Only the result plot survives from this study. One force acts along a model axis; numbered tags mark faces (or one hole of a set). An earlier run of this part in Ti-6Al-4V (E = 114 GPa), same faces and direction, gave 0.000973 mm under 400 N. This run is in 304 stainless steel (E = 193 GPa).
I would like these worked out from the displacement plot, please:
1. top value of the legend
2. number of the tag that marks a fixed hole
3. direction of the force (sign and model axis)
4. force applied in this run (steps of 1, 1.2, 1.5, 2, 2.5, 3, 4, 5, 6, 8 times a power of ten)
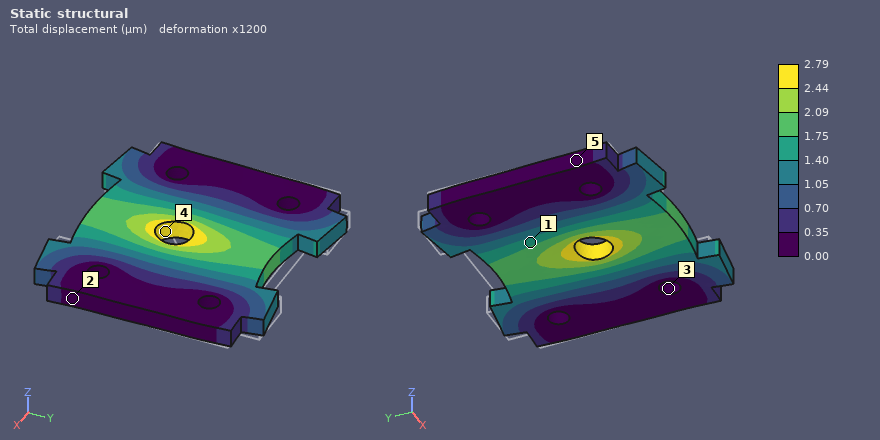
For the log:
2.79 µm
3
-Y
2 kN
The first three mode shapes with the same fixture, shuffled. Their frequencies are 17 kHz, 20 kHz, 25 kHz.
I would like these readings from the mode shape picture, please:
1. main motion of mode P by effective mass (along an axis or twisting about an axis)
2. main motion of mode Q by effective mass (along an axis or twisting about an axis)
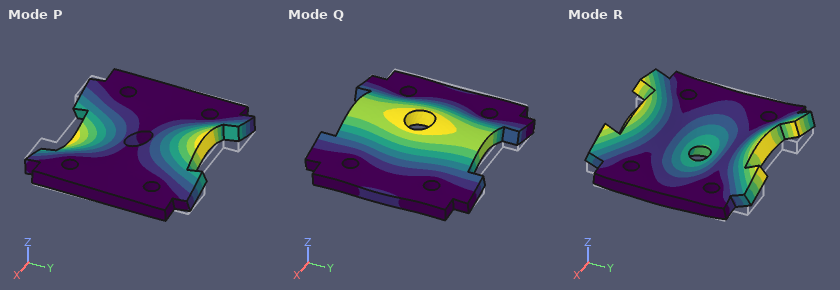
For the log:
twisting about X
along Z
